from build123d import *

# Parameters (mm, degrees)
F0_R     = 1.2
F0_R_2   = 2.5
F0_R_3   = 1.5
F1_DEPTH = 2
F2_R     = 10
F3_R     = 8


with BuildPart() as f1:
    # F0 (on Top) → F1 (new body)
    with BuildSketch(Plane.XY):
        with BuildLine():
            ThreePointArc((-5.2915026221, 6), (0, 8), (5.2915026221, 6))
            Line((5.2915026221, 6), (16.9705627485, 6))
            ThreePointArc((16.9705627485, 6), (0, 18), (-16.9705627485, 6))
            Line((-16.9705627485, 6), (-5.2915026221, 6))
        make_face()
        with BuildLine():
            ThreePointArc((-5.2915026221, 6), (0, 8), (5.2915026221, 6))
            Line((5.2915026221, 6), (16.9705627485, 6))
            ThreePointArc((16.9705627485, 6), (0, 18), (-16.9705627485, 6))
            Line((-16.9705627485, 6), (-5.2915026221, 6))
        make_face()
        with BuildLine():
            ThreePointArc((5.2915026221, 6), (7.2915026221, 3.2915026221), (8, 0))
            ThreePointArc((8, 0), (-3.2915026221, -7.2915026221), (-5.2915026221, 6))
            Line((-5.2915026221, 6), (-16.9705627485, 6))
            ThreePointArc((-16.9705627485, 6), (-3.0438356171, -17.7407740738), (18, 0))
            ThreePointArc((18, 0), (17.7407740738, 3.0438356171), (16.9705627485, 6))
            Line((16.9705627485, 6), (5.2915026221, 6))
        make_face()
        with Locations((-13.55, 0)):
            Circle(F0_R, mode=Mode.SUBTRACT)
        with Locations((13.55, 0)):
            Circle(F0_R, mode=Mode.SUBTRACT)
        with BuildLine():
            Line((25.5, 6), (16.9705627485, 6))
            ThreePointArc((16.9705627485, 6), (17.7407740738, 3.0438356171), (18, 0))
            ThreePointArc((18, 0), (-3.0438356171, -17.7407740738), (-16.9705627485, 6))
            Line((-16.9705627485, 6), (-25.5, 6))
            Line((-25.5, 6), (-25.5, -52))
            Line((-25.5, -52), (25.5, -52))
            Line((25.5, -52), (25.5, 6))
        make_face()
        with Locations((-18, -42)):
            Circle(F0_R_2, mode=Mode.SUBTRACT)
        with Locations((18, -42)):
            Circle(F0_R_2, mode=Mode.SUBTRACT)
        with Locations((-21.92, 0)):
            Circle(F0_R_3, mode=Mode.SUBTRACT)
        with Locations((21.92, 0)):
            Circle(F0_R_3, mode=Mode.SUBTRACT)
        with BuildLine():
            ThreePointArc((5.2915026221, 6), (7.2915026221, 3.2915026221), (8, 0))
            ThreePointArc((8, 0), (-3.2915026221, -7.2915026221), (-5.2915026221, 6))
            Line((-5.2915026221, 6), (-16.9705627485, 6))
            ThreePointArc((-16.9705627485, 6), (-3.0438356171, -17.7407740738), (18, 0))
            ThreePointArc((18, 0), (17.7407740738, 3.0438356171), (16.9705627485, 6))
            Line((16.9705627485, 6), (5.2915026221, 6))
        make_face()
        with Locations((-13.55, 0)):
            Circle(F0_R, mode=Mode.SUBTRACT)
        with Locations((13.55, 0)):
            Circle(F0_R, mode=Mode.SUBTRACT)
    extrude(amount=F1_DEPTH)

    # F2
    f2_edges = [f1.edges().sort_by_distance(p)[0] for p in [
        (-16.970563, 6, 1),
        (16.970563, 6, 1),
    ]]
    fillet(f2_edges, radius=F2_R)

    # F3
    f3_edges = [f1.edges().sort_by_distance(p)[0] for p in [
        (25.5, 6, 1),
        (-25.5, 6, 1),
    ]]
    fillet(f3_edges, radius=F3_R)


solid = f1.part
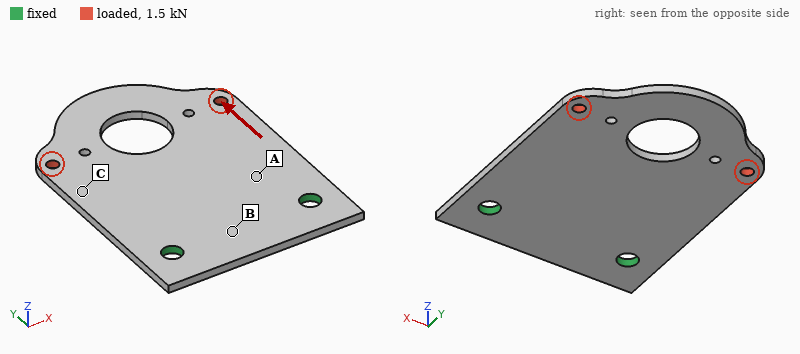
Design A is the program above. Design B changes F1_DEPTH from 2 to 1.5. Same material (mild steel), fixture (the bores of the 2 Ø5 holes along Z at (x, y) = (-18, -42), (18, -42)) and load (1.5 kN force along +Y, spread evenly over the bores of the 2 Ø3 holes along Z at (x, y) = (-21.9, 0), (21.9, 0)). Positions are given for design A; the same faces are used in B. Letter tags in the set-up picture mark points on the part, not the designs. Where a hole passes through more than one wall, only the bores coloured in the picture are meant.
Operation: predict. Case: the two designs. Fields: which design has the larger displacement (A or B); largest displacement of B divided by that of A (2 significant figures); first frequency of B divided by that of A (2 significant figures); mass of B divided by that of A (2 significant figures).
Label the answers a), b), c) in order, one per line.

a) B
b) 1.3
c) 0.75
d) 0.75
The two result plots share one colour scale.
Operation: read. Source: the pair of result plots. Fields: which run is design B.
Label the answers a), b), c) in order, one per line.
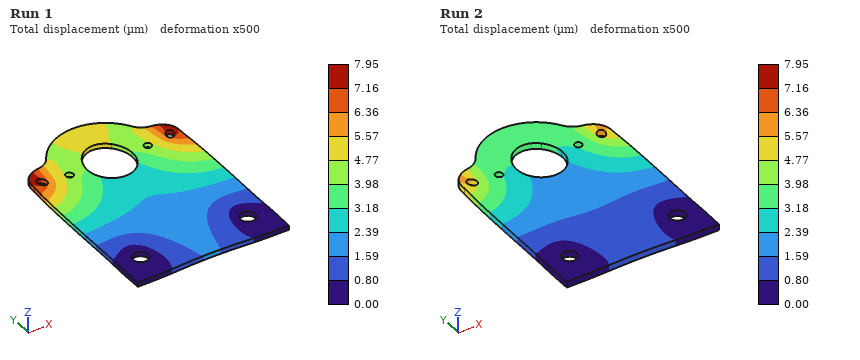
a) Run 1
